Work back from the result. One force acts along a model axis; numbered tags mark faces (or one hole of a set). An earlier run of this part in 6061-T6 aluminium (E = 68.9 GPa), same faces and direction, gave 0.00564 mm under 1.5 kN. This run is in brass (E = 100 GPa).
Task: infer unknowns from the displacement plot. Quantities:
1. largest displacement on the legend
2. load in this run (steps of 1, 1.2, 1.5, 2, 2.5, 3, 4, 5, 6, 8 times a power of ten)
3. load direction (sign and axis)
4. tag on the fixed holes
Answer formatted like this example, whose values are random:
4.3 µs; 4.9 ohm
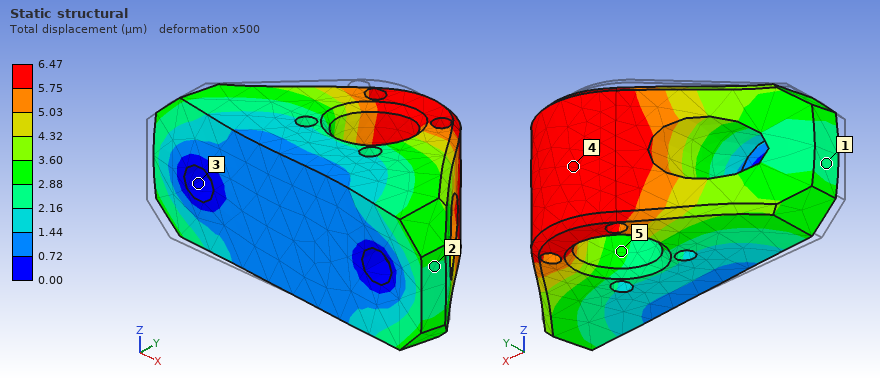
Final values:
6.47 µm; 2.5 kN; +X; 3
